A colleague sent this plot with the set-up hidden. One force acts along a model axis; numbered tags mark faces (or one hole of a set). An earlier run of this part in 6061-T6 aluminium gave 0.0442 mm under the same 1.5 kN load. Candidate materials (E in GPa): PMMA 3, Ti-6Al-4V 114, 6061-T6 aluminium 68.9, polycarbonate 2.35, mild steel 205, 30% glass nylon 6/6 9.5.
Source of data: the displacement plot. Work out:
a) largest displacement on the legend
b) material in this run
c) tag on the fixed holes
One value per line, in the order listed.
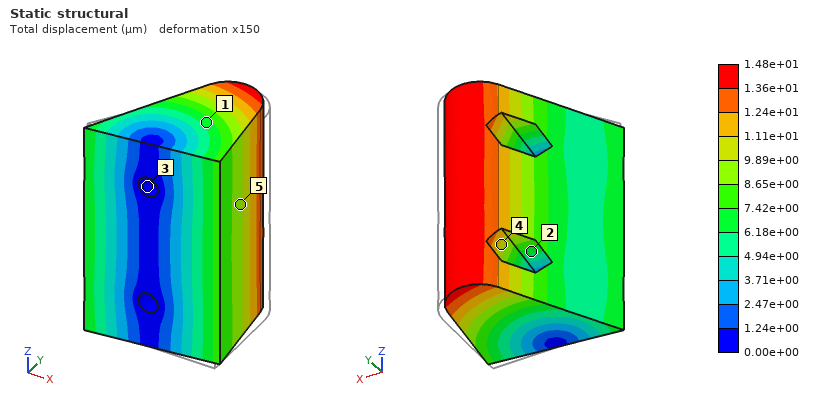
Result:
1.48e+01 µm
mild steel
3
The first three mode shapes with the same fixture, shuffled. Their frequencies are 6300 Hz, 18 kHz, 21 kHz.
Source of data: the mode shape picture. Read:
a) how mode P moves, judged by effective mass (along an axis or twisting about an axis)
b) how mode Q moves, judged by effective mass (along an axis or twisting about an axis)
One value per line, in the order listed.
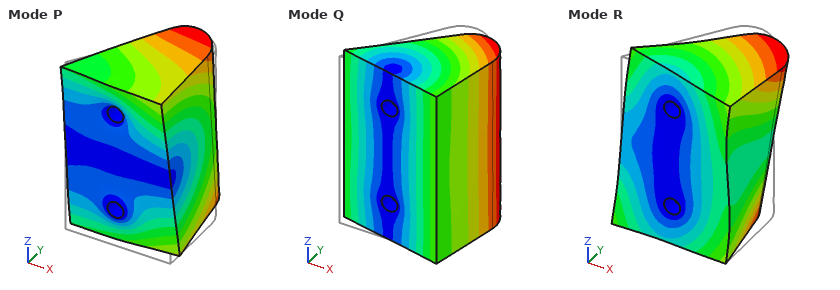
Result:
along Z
along X
